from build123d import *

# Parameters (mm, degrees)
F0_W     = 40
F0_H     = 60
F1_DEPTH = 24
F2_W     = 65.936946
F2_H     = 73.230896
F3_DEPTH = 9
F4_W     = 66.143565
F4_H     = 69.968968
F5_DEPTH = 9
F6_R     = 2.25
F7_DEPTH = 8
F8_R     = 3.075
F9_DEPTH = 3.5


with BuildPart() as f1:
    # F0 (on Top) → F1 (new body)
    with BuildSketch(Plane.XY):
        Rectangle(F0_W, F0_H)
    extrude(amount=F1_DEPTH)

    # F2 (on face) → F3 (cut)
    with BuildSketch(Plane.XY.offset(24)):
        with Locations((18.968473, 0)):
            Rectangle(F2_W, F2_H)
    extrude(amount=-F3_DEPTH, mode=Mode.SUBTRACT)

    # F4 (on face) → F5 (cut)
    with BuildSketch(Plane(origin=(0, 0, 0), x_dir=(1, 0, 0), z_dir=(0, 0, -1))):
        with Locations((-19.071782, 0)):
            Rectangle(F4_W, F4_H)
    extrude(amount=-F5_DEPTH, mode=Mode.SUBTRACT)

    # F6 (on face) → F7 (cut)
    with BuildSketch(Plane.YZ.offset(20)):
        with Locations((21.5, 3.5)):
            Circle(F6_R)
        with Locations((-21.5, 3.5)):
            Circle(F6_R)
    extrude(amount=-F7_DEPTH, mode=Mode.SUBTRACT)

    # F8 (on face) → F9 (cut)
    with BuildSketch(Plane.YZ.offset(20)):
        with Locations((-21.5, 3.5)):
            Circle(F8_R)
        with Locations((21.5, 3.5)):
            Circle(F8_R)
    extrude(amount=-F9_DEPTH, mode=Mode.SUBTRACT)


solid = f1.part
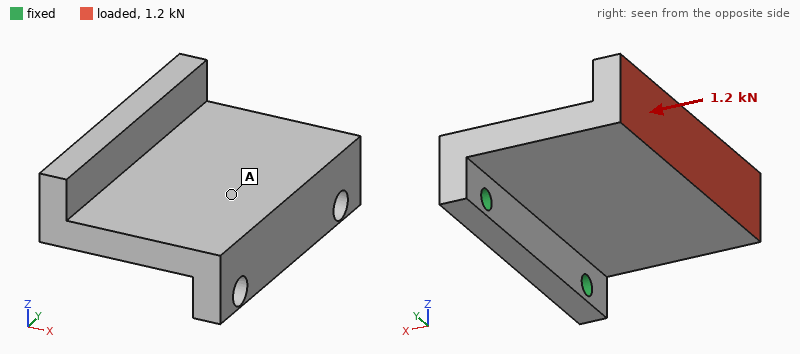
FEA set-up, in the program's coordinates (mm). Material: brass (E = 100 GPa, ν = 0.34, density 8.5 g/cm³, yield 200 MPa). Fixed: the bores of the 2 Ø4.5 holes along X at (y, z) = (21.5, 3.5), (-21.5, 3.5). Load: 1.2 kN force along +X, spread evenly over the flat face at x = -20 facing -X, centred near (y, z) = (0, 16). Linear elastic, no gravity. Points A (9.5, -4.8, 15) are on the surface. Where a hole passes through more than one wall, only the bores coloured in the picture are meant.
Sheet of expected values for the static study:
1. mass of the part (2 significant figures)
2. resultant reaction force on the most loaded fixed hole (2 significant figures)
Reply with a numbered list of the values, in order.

1. 180 g
2. 600 N
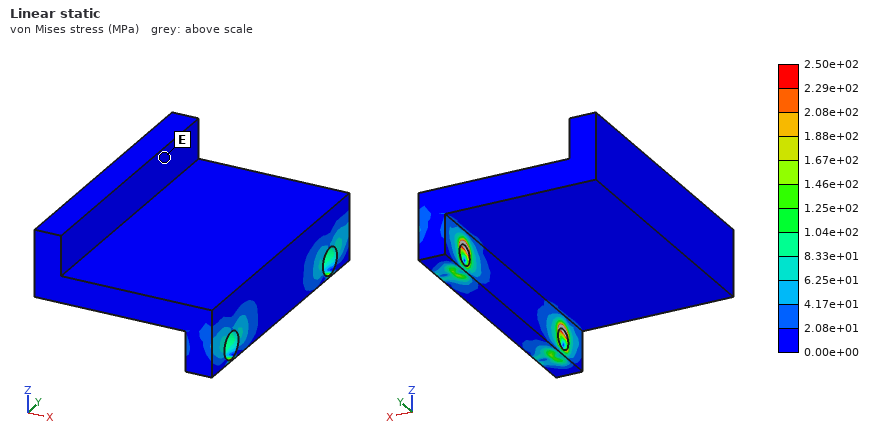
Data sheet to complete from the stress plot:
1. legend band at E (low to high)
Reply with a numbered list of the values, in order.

1. 0.00e+00 to 2.08e+01 MPa
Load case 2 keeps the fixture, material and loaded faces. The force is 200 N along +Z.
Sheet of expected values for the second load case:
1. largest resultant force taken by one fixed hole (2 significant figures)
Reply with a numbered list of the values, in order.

1. 100 N
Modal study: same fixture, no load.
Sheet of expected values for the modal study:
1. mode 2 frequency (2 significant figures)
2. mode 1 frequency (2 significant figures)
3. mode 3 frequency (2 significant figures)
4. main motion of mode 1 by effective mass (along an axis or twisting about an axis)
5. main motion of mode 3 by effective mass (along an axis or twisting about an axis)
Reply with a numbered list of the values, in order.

1. 2700 Hz
2. 900 Hz
3. 4000 Hz
4. along Z
5. along Y
